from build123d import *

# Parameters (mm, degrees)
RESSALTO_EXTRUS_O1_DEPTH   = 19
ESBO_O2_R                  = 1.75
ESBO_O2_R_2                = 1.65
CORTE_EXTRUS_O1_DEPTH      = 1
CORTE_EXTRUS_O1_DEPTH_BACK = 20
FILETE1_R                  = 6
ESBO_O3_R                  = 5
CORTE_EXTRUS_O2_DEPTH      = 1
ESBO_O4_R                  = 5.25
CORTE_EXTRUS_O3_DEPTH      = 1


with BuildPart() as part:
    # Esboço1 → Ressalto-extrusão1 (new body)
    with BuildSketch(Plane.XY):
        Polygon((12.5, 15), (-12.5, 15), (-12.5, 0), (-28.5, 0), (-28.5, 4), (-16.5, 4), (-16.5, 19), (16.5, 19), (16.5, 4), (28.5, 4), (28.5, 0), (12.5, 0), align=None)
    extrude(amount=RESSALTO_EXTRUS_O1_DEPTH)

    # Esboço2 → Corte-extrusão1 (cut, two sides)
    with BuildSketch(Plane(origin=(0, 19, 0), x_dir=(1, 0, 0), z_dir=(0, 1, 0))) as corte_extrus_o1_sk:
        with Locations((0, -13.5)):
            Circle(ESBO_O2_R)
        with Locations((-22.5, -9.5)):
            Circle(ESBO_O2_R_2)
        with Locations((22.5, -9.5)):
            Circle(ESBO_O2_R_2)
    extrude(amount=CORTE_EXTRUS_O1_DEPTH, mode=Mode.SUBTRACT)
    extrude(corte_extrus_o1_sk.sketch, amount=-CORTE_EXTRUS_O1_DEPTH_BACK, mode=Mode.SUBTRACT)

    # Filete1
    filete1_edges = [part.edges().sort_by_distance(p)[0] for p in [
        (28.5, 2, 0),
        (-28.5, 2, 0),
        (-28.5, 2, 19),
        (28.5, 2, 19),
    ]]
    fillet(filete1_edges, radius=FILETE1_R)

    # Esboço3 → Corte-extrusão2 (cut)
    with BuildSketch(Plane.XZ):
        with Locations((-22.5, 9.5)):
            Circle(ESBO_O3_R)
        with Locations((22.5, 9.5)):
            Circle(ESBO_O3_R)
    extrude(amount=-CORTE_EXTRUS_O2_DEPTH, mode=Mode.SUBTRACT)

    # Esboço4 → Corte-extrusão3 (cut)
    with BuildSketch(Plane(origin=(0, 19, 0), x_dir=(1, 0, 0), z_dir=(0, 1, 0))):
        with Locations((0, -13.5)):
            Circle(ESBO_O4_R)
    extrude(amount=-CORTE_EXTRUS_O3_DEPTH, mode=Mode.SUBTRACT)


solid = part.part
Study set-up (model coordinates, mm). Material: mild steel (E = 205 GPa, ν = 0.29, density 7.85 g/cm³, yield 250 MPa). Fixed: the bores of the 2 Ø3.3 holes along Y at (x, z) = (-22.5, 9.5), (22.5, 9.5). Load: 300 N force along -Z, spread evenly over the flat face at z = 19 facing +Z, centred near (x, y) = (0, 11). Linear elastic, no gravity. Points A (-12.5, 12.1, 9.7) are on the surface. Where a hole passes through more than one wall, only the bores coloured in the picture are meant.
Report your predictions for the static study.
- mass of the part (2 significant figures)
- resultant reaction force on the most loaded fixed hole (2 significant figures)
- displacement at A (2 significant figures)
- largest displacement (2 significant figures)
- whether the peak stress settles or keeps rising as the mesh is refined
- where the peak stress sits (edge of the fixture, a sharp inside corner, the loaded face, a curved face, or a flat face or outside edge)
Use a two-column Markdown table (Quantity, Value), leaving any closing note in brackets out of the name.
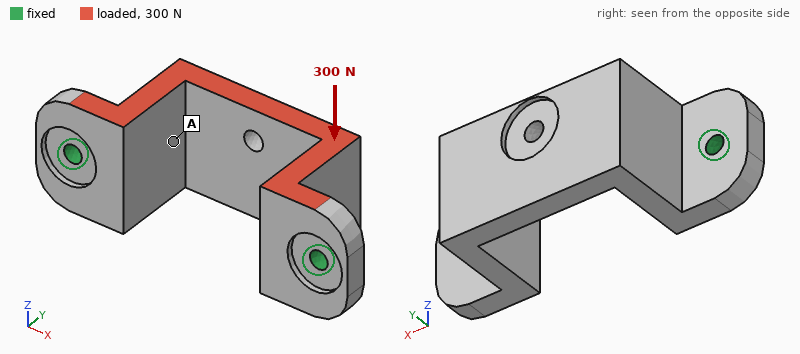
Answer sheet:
| Quantity | Value |
|---|---|
| mass of the part | 48 g |
| resultant reaction force on the most loaded fixed hole | 150 N |
| displacement at A | 5.9 µm |
| largest displacement | 11 µm |
| whether the peak stress settles or keeps rising as the mesh is refined | keeps rising |
| where the peak stress sits | edge of the fixture |
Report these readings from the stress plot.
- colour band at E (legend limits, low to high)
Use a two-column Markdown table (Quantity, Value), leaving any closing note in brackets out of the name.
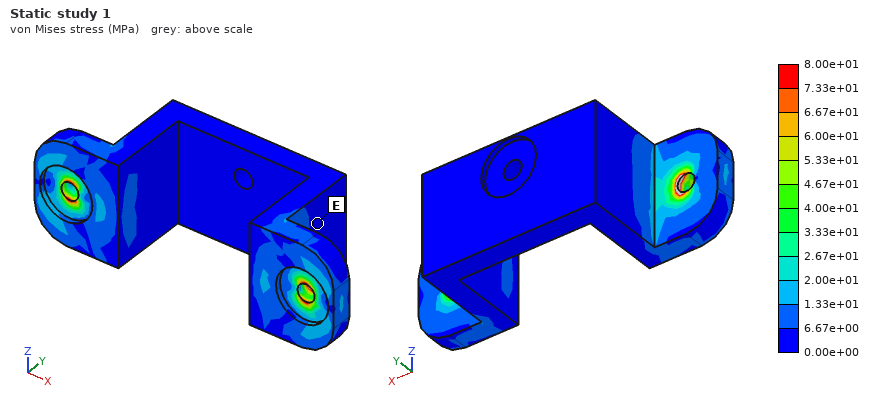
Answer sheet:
| Quantity | Value |
|---|---|
| colour band at E | 0.00e+00 to 6.67e+00 MPa |
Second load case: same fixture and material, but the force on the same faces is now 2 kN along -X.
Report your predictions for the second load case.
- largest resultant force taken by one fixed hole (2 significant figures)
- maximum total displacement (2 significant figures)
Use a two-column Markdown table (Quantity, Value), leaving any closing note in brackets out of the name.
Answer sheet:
| Quantity | Value |
|---|---|
| largest resultant force taken by one fixed hole | 1.1 kN |
| maximum total displacement | 36 µm |
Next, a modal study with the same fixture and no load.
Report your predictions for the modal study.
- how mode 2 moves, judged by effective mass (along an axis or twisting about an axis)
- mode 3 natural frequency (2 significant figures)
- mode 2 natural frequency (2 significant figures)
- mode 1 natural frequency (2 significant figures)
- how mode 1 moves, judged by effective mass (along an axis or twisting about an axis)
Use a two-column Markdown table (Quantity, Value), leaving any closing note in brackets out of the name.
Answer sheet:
| Quantity | Value |
|---|---|
| how mode 2 moves, judged by effective mass | along X |
| mode 3 natural frequency | 9200 Hz |
| mode 2 natural frequency | 7600 Hz |
| mode 1 natural frequency | 4500 Hz |
| how mode 1 moves, judged by effective mass | along Z |
